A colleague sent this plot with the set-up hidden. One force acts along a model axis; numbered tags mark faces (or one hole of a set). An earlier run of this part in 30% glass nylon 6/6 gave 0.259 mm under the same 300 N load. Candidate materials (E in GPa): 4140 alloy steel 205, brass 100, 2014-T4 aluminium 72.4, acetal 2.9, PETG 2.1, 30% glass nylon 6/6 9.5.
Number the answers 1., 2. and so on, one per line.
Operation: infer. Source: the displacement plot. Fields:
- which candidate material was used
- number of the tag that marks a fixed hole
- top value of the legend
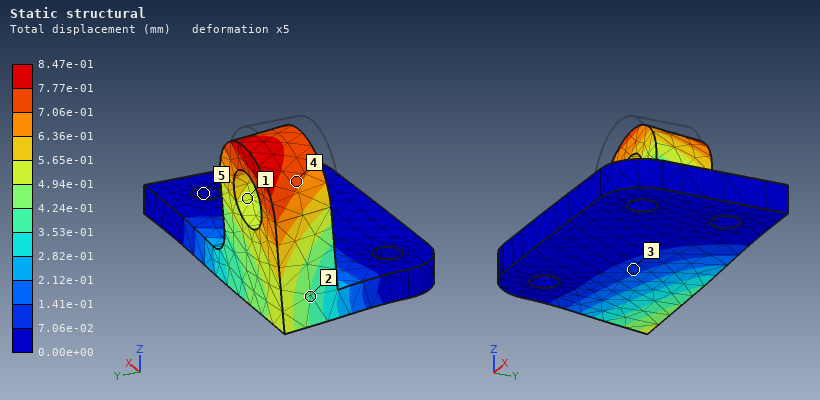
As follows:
1. acetal
2. 5
3. 8.47e-01 mm
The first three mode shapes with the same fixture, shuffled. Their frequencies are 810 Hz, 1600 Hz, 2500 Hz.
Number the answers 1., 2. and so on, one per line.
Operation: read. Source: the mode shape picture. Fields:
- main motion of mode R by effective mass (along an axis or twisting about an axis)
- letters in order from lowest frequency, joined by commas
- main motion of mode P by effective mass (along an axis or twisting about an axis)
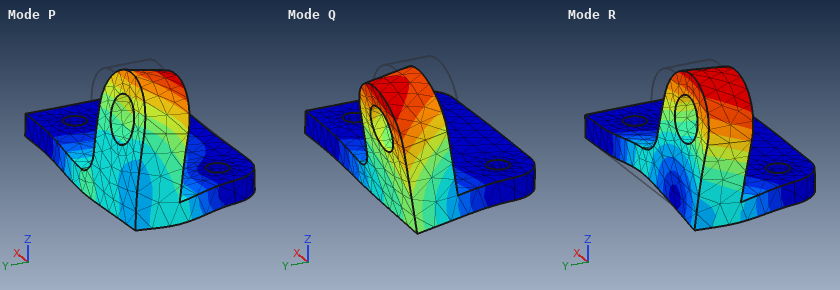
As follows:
1. along X
2. Q, R, P
3. along Z
